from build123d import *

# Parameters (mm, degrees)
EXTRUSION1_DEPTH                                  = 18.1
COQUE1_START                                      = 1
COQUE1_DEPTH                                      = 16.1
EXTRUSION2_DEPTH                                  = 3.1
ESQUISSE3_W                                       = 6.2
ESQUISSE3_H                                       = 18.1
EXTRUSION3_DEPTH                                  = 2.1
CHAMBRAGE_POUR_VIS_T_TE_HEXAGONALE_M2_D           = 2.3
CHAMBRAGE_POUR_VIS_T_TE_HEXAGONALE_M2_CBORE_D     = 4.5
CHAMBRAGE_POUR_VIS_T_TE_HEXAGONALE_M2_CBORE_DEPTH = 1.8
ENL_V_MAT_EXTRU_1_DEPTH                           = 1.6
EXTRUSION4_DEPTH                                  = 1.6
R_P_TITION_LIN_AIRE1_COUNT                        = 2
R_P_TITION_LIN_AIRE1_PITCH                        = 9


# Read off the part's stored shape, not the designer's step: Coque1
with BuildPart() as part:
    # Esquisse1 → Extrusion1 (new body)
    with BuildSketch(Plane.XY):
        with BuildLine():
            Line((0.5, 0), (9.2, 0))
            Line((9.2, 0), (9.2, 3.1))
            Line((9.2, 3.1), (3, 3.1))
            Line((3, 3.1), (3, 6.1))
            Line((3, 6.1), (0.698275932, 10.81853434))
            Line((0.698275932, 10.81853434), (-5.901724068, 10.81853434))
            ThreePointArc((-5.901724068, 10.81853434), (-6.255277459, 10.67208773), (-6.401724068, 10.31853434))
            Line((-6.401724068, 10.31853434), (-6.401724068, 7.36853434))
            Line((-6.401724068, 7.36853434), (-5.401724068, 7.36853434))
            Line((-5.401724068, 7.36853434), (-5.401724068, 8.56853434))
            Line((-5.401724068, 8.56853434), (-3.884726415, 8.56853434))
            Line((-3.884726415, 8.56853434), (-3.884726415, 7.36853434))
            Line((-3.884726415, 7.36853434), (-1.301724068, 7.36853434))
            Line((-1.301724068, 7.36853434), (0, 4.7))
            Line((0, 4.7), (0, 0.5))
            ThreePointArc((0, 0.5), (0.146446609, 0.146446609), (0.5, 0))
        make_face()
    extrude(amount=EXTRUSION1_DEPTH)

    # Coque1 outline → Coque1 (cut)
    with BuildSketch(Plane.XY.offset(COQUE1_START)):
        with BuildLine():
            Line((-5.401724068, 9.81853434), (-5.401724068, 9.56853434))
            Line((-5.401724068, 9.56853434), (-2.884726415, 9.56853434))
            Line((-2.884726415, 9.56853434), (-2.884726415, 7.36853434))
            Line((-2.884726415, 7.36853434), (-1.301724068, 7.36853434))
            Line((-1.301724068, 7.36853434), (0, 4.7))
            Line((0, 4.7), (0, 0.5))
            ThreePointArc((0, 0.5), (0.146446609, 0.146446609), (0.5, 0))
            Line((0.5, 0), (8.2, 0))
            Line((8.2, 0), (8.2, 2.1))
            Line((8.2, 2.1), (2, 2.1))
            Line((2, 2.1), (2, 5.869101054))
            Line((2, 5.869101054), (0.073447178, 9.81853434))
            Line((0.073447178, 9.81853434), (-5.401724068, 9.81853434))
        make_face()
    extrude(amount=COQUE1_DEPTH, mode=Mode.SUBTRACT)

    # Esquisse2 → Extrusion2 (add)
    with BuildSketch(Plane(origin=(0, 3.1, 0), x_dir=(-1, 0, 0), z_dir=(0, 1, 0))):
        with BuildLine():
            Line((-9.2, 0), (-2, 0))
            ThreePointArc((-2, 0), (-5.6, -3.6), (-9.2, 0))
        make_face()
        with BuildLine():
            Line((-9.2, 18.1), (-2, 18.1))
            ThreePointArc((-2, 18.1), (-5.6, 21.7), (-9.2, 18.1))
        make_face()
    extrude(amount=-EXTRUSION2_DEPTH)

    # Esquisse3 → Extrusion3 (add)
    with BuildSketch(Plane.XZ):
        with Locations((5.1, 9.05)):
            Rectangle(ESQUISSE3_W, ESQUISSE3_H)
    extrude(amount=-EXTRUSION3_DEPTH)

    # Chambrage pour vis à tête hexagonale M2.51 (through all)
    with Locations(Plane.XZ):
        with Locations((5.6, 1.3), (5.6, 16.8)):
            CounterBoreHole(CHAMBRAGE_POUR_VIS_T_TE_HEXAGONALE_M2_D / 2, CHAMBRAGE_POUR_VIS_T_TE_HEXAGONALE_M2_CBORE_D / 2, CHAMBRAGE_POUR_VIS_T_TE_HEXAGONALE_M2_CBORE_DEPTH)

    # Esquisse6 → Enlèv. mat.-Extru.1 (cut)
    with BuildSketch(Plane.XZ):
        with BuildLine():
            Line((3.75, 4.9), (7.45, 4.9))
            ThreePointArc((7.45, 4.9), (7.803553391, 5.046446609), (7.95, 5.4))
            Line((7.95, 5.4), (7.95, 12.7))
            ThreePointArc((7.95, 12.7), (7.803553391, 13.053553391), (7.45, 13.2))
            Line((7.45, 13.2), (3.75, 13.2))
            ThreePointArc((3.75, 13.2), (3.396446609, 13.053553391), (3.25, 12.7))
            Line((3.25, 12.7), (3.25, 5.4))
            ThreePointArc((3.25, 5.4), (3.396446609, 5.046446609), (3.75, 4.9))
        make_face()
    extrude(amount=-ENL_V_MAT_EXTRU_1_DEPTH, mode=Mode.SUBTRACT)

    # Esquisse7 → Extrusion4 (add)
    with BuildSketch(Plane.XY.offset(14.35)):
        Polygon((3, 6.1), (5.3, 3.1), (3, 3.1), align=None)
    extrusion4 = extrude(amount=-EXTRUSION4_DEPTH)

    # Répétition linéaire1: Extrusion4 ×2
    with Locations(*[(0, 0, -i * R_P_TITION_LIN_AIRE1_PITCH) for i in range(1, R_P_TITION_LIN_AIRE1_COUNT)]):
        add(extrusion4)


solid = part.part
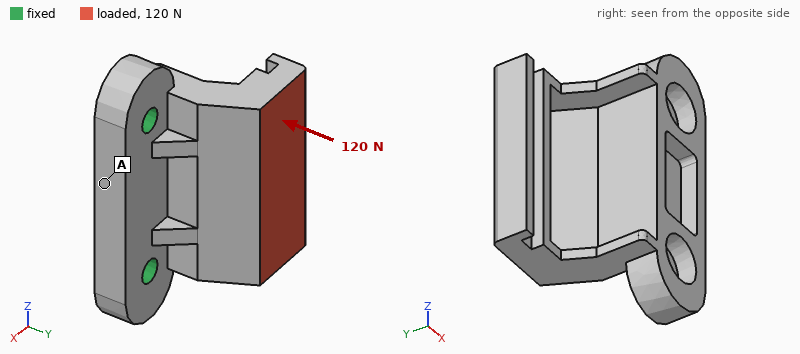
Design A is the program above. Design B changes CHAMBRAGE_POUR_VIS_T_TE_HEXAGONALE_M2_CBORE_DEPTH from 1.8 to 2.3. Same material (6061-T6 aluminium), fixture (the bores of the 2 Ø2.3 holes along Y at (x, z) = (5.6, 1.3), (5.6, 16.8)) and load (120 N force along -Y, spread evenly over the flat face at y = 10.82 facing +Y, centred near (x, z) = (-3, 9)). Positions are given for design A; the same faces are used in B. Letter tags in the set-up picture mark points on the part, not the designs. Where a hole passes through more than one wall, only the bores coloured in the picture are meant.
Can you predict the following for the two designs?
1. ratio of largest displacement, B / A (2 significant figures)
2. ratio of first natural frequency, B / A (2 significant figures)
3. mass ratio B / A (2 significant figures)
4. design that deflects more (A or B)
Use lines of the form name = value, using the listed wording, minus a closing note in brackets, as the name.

ratio of largest displacement, B / A = 1.4
ratio of first natural frequency, B / A = 0.85
mass ratio B / A = 0.99
design that deflects more = B
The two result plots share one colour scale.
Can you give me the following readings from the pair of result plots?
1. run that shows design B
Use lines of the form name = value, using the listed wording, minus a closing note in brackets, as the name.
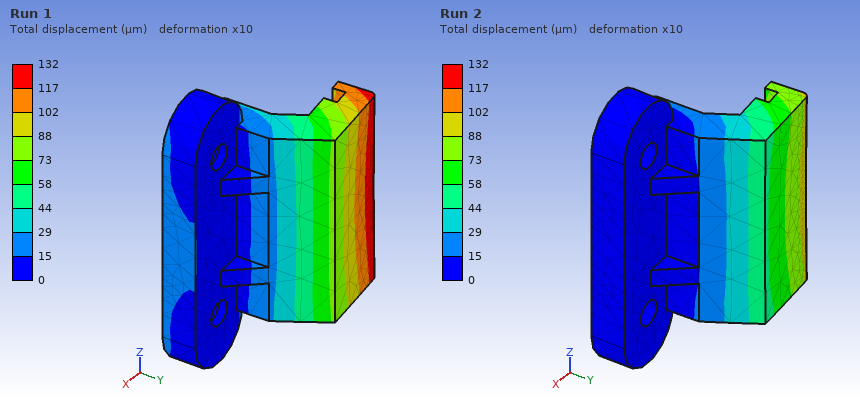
run that shows design B = Run 1
